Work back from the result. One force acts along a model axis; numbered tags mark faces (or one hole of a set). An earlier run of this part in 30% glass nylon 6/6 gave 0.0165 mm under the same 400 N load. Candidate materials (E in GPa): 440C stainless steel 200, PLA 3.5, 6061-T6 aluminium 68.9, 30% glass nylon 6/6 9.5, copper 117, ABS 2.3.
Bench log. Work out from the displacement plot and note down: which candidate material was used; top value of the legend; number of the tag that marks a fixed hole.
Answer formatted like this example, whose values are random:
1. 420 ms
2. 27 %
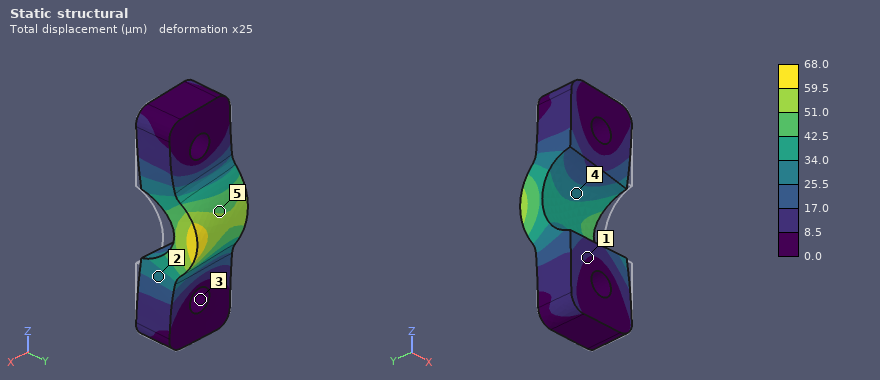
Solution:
1. ABS
2. 68.0 µm
3. 3
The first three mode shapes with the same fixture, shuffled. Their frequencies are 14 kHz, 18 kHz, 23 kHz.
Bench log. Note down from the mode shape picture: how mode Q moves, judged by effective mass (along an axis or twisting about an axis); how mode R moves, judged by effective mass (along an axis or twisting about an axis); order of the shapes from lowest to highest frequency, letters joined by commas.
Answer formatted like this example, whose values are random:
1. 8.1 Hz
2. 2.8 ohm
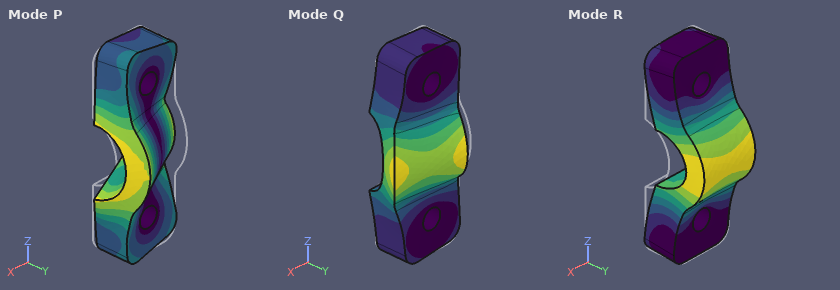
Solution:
1. along X
2. along Y
3. Q, R, P
